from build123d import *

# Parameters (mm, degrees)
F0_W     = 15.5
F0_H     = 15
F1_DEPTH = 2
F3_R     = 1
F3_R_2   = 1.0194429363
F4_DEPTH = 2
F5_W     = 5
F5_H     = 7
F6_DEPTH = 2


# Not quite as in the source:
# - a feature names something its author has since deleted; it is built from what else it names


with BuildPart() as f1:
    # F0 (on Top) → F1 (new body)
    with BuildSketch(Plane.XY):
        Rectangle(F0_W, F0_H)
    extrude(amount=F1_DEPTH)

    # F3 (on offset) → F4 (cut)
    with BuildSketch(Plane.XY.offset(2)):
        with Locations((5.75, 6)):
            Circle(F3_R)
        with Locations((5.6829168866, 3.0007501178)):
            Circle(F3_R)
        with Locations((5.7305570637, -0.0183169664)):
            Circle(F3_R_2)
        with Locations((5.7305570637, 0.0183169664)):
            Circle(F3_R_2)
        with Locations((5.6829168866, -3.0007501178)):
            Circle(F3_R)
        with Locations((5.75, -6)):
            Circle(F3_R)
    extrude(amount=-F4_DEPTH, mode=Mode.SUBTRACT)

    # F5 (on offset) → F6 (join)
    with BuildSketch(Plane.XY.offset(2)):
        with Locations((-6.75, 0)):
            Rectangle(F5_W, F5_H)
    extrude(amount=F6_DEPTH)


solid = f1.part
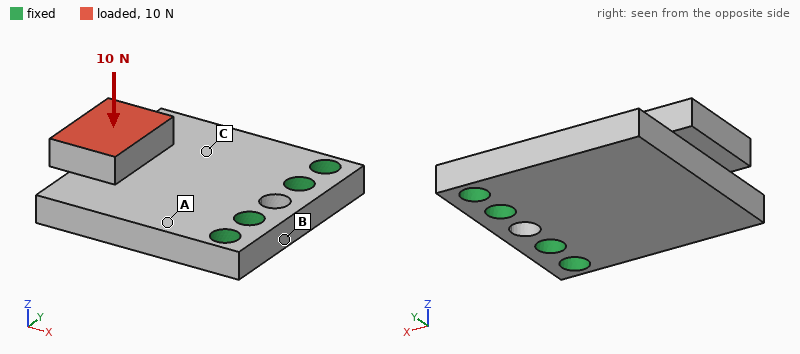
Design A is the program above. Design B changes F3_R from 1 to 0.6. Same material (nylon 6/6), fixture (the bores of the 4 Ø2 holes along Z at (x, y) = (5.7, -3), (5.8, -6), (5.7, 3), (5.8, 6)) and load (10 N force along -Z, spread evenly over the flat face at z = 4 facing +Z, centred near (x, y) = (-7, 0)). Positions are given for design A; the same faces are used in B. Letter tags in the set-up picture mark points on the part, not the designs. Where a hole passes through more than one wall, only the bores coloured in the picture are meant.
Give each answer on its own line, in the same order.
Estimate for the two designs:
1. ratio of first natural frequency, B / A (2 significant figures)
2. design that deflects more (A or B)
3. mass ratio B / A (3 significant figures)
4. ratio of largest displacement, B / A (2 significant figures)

0.92
B
1.03
1.1
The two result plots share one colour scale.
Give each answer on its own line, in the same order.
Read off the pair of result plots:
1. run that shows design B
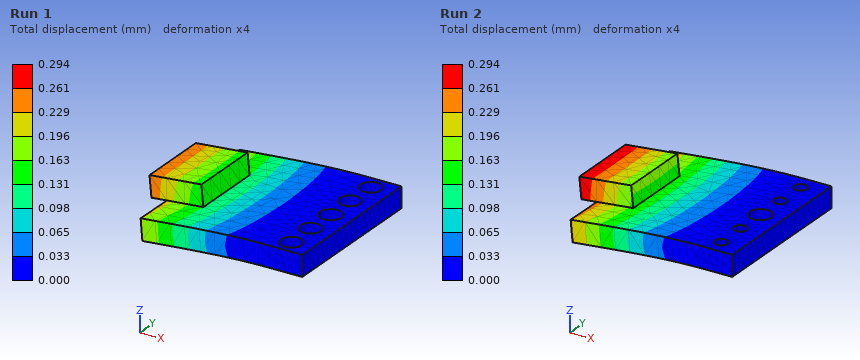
Run 2
